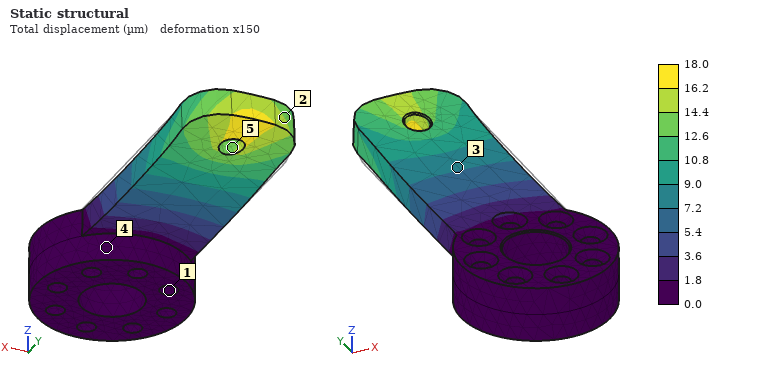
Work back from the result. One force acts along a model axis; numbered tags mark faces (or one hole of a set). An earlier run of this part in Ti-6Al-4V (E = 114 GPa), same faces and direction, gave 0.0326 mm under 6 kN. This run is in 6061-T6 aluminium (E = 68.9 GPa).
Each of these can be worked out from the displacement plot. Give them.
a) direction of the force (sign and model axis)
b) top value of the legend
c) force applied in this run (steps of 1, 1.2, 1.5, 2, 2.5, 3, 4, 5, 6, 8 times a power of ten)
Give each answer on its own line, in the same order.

+Y
18.0 µm
2 kN
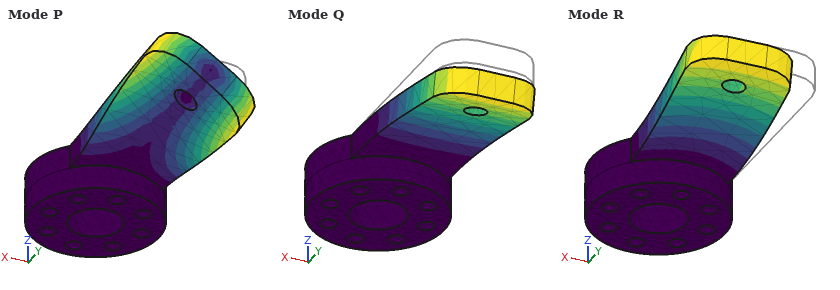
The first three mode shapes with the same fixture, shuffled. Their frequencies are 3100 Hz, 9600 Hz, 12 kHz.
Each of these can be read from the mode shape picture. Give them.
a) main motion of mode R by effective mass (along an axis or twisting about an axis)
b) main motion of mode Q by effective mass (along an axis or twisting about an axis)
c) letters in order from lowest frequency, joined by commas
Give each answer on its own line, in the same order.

along X
along Z
Q, R, P
